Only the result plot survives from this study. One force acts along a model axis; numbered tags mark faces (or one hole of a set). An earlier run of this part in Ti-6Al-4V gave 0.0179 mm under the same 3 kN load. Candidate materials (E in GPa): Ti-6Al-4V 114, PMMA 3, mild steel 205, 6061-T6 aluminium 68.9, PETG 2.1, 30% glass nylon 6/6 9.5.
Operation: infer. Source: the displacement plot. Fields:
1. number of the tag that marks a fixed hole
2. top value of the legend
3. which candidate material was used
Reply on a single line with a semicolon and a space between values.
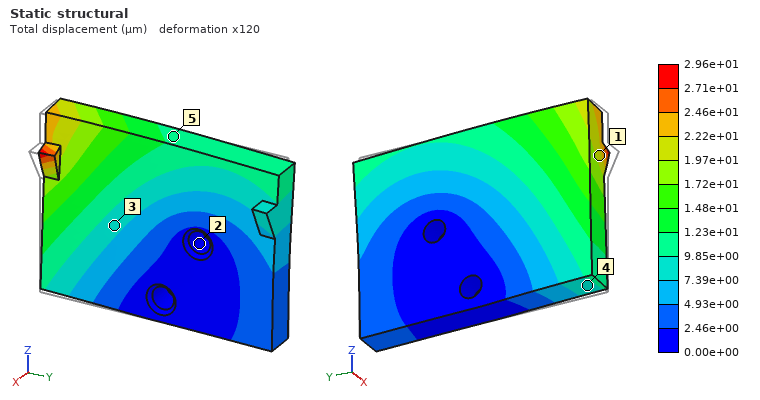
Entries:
2; 2.96e+01 µm; 6061-T6 aluminium
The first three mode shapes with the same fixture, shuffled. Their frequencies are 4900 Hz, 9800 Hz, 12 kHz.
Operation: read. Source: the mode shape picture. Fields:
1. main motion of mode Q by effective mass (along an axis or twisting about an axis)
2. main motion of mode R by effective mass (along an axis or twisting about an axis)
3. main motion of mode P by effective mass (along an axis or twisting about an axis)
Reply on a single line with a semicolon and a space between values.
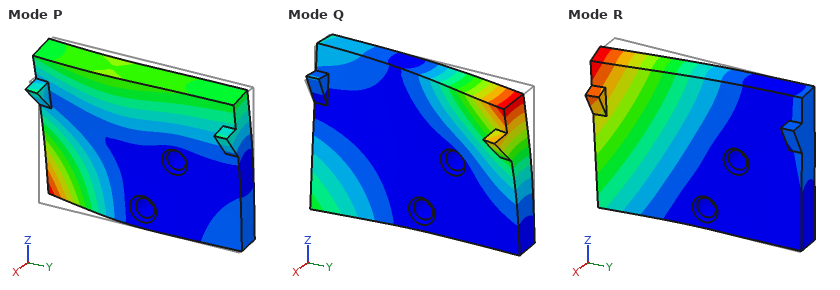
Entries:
along X; along X; twisting about Y
